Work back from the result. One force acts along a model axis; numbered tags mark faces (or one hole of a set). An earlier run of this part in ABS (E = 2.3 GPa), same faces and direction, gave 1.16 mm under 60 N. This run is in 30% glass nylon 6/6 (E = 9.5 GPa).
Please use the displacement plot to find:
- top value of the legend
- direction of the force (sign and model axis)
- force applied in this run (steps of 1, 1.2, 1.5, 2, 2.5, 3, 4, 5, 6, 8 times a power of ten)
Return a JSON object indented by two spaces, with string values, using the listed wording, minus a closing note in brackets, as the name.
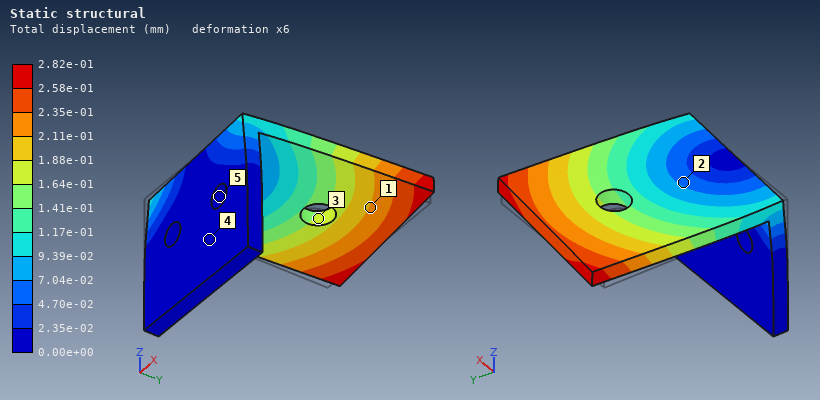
{
  "top value of the legend": "2.82e-01 mm",
  "direction of the force": "+X",
  "force applied in this run": "60 N"
}
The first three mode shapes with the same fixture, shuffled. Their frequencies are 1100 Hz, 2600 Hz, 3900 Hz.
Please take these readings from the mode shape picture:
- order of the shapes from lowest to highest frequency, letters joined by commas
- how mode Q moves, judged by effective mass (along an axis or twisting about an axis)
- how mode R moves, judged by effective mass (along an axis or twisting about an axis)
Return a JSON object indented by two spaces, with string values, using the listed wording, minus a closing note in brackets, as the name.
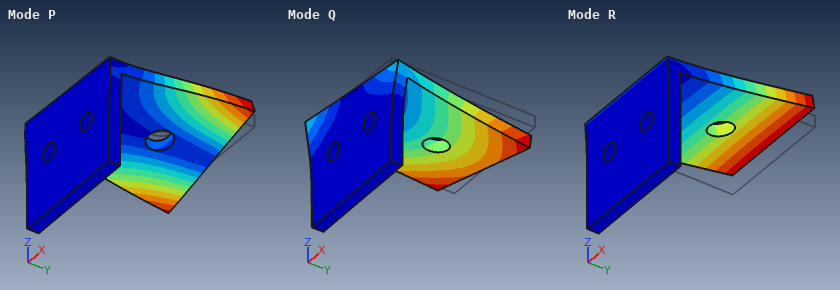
{
  "order of the shapes from lowest to highest frequency, letters joined by commas": "R, Q, P",
  "how mode Q moves, judged by effective mass": "along X",
  "how mode R moves, judged by effective mass": "along Z"
}
